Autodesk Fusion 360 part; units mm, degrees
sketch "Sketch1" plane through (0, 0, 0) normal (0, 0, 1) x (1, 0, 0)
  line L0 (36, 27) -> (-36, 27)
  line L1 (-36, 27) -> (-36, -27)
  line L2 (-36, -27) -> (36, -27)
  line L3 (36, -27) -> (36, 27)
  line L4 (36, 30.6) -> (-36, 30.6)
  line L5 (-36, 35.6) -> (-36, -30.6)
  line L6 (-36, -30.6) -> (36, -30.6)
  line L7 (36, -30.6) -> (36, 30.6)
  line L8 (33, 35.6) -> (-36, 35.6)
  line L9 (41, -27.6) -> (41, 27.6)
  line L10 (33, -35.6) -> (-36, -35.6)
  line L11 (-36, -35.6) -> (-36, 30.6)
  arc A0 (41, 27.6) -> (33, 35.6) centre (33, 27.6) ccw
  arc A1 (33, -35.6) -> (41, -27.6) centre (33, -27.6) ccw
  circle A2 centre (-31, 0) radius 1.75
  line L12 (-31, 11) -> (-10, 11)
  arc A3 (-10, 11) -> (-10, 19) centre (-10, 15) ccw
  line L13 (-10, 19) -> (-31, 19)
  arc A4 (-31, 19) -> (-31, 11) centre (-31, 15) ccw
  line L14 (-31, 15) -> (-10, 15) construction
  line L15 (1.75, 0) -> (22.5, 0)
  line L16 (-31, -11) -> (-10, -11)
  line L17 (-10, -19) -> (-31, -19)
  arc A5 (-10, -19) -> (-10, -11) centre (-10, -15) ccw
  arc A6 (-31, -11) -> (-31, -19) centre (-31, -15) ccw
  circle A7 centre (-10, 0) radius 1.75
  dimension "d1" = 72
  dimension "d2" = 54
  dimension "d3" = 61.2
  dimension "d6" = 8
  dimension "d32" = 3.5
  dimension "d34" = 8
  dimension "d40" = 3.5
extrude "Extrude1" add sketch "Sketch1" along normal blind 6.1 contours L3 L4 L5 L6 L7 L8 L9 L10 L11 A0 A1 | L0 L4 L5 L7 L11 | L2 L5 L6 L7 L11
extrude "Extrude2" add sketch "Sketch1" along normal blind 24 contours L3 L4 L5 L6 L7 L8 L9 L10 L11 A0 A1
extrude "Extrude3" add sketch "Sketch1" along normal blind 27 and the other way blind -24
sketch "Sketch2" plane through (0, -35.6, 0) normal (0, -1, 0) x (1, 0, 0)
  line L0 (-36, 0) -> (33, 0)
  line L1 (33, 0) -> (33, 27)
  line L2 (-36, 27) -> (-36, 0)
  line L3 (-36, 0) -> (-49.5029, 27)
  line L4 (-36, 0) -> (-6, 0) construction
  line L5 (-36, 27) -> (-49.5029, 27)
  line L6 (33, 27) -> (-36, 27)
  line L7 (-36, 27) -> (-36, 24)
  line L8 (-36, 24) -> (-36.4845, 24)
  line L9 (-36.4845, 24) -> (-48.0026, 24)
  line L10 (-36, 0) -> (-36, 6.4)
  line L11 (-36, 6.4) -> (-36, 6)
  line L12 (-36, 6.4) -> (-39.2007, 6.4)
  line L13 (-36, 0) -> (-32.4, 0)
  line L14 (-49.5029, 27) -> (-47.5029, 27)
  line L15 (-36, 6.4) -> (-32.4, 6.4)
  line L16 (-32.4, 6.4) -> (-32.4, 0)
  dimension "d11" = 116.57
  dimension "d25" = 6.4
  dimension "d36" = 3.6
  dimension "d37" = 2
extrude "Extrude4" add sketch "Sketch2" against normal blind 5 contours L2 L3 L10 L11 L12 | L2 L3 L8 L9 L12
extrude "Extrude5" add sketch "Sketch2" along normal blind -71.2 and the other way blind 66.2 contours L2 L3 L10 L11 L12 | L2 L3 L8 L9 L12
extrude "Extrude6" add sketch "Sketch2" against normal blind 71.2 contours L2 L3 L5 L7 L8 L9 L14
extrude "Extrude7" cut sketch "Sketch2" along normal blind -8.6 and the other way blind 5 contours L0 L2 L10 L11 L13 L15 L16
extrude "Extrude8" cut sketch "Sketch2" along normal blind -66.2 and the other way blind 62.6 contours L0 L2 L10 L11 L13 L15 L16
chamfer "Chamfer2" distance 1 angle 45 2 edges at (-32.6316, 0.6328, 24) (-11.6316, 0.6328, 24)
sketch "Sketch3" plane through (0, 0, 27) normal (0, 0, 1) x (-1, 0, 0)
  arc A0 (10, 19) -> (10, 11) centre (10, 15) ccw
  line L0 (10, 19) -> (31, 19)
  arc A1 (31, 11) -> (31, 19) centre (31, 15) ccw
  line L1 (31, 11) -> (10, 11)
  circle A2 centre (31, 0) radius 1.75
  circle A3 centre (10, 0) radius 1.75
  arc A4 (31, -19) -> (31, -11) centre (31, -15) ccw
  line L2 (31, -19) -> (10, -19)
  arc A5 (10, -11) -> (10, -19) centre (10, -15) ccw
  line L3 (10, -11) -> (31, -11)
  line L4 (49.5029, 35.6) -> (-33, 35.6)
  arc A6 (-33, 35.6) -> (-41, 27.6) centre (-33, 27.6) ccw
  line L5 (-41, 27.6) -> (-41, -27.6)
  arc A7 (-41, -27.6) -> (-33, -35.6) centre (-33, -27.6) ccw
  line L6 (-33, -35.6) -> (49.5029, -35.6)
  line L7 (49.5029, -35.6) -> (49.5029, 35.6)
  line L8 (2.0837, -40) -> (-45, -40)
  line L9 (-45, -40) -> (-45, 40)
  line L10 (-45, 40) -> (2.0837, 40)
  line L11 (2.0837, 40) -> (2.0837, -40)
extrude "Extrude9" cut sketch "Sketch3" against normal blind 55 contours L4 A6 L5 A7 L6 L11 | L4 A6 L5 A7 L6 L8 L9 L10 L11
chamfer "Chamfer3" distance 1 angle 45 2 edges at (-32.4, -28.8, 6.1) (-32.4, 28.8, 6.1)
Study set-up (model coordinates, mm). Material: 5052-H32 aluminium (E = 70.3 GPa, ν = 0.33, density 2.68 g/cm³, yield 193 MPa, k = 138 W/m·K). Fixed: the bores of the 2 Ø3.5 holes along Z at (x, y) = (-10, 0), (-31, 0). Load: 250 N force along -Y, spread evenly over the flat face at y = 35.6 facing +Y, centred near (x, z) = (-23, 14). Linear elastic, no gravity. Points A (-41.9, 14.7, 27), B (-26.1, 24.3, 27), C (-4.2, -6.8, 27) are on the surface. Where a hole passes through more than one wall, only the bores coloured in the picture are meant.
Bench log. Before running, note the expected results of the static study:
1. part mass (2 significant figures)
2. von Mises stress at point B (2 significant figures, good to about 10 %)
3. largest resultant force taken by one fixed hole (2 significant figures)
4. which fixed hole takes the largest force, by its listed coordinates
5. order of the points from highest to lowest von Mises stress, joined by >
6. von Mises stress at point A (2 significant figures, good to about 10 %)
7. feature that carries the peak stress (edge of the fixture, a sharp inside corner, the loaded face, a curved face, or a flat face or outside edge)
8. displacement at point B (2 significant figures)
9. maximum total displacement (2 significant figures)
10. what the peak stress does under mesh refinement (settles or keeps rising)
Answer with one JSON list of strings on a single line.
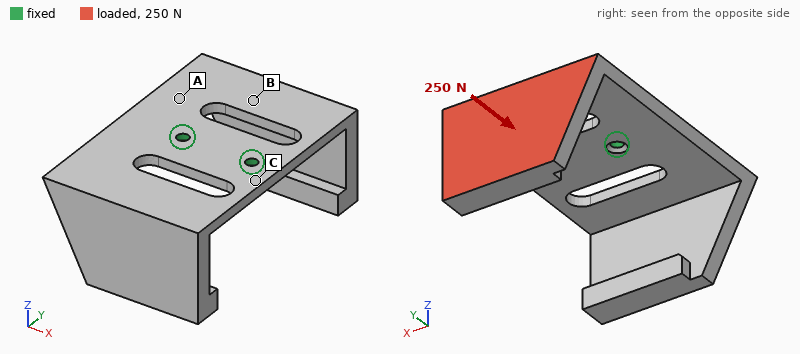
["52 g", "25 MPa", "150 N", "(-31, 0)", "A > B > C", "83 MPa", "edge of the fixture", "0.24 mm", "0.79 mm", "keeps rising"]
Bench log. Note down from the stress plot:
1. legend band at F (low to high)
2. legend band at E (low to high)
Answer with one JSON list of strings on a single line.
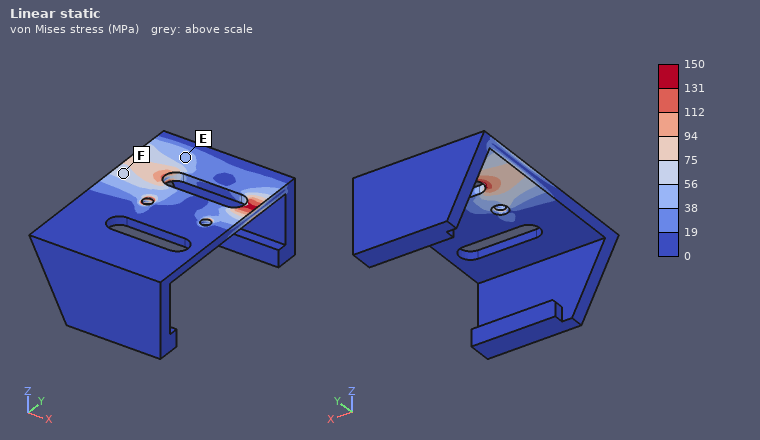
["56 to 75 MPa", "38 to 56 MPa"]
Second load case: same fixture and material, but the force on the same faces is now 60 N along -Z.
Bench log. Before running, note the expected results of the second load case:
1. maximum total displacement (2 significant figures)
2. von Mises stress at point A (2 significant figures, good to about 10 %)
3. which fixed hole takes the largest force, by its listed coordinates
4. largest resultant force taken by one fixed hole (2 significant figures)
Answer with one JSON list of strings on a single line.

["0.37 mm", "38 MPa", "(-31, 0)", "34 N"]
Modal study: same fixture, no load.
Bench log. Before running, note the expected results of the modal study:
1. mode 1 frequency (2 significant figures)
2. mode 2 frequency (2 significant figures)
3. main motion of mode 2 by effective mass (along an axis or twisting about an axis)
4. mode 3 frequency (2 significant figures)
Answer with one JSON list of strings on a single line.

["500 Hz", "580 Hz", "along Z", "1300 Hz"]
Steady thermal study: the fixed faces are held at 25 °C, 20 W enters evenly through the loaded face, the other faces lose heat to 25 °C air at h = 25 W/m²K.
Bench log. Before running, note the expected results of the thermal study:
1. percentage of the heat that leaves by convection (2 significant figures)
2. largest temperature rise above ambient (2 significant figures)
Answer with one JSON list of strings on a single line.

["26 %", "61 K"]
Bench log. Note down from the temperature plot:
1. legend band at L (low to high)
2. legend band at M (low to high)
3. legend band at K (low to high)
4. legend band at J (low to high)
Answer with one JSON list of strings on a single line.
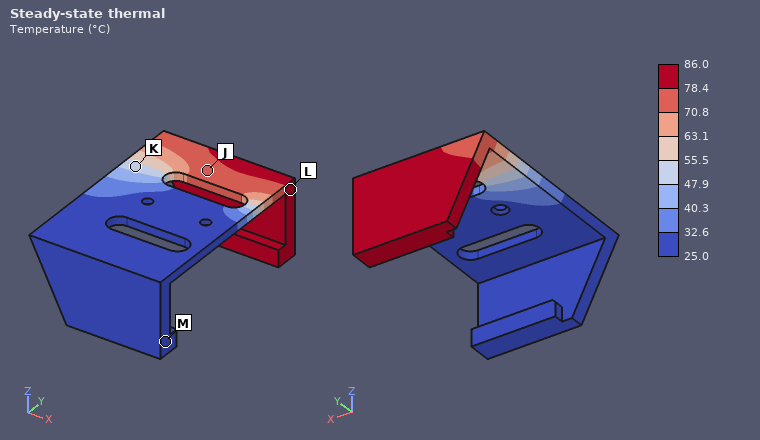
["78.4 to 86.0 °C", "25.0 to 32.6 °C", "47.9 to 55.5 °C", "70.8 to 78.4 °C"]
